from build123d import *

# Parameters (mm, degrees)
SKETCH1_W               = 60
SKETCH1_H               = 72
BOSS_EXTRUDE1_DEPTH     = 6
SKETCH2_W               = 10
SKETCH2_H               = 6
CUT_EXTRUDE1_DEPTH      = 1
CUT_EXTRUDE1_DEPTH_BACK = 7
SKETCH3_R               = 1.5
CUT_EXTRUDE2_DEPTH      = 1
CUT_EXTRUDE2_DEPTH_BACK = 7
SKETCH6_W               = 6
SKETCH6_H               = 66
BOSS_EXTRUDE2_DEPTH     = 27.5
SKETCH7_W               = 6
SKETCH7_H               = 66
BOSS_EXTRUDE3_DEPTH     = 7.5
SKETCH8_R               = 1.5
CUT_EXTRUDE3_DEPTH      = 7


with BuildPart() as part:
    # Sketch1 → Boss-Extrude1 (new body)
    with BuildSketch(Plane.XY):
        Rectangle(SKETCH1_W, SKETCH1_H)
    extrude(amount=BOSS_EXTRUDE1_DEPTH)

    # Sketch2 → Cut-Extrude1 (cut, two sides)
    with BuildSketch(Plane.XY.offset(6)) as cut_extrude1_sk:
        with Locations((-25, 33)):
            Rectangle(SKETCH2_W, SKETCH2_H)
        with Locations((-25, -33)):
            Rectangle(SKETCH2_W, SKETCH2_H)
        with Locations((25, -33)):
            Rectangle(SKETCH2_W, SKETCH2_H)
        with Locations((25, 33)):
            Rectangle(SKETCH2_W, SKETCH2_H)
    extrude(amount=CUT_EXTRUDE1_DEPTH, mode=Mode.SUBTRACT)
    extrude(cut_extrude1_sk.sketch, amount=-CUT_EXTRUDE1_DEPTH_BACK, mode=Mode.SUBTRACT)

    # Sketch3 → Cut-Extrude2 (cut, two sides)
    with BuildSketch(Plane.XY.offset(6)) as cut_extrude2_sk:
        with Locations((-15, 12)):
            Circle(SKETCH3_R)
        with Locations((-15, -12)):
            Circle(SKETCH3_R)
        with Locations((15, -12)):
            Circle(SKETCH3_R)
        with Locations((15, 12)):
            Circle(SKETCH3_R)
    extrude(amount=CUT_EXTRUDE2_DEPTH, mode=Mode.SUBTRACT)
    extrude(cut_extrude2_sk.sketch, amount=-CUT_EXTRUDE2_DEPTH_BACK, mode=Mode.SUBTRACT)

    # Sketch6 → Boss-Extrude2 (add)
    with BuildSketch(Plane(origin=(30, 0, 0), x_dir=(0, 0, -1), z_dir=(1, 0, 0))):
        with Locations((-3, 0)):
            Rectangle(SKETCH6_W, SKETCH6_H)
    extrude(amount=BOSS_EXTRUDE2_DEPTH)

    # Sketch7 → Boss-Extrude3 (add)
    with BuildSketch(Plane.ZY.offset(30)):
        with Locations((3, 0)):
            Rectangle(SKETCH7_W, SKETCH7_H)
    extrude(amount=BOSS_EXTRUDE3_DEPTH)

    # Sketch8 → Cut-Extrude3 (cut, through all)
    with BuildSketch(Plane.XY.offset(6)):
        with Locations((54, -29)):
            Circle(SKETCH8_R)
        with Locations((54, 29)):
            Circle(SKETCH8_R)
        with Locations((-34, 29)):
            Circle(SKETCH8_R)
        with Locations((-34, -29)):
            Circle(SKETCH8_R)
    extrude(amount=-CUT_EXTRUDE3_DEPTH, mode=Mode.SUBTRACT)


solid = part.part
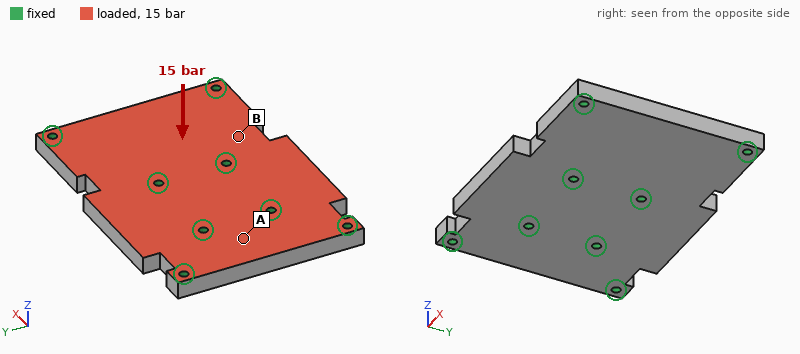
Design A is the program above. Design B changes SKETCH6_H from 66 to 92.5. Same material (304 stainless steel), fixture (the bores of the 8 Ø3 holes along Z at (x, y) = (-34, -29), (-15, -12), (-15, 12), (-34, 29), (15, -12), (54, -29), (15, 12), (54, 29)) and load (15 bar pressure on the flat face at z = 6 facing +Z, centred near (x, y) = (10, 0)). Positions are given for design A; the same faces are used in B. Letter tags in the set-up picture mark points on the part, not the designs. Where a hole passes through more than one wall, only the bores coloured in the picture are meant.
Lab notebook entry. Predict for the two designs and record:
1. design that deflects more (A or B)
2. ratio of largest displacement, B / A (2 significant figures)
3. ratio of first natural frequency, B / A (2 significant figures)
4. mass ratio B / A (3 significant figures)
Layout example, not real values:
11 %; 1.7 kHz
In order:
B; 1.4; 0.91; 1.12
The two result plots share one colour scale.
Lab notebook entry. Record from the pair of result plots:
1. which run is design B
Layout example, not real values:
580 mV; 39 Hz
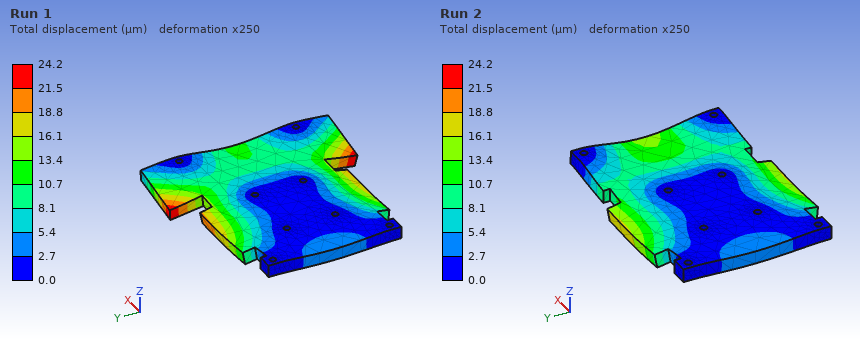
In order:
Run 1
